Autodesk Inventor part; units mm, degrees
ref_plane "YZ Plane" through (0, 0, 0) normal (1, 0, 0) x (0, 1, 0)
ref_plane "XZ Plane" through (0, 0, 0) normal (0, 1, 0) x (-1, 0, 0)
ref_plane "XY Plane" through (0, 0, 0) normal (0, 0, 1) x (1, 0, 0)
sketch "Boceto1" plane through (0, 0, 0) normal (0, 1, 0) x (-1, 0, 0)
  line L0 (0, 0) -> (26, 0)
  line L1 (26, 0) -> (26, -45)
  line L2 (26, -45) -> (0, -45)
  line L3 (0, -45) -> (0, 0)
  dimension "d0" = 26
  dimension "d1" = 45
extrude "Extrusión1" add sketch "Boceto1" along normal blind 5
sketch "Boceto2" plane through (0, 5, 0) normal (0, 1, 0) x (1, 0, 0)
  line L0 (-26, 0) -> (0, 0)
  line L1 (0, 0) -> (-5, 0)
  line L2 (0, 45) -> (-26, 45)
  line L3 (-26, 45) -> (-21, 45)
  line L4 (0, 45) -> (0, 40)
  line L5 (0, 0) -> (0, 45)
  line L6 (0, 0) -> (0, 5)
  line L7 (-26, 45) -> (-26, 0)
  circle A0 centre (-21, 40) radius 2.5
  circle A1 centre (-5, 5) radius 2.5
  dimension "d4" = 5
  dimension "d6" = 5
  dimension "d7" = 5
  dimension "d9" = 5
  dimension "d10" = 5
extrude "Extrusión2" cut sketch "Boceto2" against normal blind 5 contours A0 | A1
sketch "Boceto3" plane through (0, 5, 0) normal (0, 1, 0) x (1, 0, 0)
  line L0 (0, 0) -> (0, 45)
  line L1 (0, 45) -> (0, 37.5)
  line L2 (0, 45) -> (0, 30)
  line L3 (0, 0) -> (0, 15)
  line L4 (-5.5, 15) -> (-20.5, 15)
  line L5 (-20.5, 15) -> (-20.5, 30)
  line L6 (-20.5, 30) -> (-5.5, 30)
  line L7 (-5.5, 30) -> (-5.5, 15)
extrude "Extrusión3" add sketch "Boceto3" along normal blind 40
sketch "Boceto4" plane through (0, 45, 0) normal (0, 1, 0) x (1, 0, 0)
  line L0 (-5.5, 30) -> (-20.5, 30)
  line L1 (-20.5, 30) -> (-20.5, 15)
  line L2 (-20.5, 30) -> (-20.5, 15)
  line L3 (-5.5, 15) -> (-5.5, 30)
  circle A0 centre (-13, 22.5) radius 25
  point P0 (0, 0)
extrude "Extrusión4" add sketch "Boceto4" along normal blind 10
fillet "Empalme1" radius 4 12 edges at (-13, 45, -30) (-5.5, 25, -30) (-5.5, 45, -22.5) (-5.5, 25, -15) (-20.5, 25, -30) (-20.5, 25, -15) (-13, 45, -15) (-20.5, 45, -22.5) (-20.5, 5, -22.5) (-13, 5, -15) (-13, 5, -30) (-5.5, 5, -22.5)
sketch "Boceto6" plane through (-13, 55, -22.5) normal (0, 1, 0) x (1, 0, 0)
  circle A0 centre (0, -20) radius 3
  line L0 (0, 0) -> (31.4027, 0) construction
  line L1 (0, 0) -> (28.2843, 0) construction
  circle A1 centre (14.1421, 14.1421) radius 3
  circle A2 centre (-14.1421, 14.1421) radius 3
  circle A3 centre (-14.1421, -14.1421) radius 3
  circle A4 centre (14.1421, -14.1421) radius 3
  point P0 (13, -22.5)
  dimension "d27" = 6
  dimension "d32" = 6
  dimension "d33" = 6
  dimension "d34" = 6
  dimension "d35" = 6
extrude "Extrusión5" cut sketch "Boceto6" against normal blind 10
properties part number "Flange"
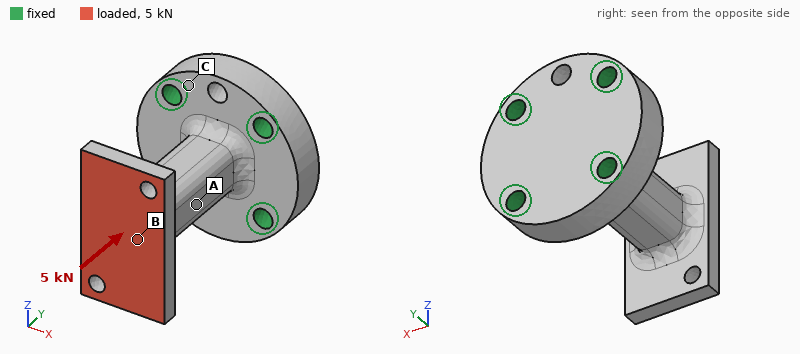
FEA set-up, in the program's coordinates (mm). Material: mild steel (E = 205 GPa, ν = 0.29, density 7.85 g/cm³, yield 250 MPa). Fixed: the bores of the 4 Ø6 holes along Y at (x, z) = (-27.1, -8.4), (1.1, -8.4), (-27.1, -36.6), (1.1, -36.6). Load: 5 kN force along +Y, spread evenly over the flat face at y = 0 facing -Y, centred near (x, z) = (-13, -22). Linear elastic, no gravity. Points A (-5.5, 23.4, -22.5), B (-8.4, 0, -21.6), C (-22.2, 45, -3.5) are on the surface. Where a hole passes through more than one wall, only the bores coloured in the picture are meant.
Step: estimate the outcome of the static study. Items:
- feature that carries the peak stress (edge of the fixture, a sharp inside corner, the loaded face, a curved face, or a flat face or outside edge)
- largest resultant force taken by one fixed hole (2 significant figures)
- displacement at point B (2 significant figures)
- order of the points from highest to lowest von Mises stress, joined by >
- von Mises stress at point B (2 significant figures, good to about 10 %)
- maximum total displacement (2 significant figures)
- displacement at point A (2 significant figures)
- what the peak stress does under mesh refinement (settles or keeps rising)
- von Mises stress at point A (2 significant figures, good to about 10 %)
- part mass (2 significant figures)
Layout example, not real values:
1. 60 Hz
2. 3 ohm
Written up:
1. a sharp inside corner
2. 1.3 kN
3. 6.0 µm
4. B > A > C
5. 51 MPa
6. 29 µm
7. 4.4 µm
8. keeps rising
9. 24 MPa
10. 260 g
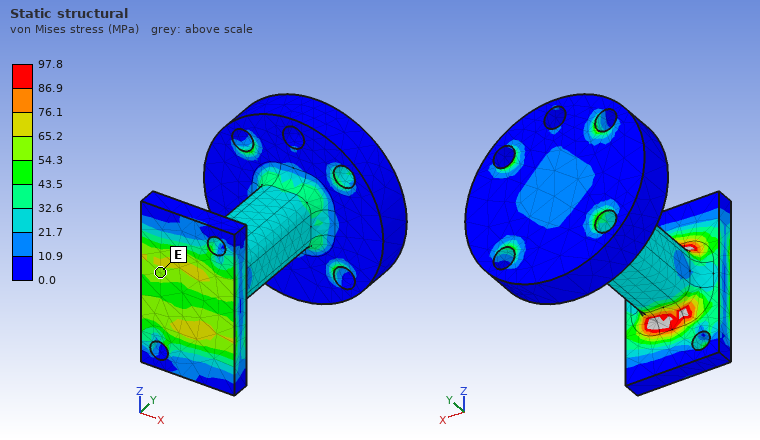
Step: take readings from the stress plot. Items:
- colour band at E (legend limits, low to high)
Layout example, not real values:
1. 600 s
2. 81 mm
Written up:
1. 54.3 to 65.2 MPa
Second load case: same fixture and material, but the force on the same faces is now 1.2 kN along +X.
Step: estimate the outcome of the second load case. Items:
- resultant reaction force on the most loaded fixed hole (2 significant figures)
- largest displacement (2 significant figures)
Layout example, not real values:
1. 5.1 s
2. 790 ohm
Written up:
1. 1.2 kN
2. 67 µm
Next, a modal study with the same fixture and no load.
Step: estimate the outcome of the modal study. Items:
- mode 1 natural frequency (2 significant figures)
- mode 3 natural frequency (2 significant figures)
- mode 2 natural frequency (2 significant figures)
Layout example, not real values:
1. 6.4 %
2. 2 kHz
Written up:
1. 2900 Hz
2. 5600 Hz
3. 3000 Hz
